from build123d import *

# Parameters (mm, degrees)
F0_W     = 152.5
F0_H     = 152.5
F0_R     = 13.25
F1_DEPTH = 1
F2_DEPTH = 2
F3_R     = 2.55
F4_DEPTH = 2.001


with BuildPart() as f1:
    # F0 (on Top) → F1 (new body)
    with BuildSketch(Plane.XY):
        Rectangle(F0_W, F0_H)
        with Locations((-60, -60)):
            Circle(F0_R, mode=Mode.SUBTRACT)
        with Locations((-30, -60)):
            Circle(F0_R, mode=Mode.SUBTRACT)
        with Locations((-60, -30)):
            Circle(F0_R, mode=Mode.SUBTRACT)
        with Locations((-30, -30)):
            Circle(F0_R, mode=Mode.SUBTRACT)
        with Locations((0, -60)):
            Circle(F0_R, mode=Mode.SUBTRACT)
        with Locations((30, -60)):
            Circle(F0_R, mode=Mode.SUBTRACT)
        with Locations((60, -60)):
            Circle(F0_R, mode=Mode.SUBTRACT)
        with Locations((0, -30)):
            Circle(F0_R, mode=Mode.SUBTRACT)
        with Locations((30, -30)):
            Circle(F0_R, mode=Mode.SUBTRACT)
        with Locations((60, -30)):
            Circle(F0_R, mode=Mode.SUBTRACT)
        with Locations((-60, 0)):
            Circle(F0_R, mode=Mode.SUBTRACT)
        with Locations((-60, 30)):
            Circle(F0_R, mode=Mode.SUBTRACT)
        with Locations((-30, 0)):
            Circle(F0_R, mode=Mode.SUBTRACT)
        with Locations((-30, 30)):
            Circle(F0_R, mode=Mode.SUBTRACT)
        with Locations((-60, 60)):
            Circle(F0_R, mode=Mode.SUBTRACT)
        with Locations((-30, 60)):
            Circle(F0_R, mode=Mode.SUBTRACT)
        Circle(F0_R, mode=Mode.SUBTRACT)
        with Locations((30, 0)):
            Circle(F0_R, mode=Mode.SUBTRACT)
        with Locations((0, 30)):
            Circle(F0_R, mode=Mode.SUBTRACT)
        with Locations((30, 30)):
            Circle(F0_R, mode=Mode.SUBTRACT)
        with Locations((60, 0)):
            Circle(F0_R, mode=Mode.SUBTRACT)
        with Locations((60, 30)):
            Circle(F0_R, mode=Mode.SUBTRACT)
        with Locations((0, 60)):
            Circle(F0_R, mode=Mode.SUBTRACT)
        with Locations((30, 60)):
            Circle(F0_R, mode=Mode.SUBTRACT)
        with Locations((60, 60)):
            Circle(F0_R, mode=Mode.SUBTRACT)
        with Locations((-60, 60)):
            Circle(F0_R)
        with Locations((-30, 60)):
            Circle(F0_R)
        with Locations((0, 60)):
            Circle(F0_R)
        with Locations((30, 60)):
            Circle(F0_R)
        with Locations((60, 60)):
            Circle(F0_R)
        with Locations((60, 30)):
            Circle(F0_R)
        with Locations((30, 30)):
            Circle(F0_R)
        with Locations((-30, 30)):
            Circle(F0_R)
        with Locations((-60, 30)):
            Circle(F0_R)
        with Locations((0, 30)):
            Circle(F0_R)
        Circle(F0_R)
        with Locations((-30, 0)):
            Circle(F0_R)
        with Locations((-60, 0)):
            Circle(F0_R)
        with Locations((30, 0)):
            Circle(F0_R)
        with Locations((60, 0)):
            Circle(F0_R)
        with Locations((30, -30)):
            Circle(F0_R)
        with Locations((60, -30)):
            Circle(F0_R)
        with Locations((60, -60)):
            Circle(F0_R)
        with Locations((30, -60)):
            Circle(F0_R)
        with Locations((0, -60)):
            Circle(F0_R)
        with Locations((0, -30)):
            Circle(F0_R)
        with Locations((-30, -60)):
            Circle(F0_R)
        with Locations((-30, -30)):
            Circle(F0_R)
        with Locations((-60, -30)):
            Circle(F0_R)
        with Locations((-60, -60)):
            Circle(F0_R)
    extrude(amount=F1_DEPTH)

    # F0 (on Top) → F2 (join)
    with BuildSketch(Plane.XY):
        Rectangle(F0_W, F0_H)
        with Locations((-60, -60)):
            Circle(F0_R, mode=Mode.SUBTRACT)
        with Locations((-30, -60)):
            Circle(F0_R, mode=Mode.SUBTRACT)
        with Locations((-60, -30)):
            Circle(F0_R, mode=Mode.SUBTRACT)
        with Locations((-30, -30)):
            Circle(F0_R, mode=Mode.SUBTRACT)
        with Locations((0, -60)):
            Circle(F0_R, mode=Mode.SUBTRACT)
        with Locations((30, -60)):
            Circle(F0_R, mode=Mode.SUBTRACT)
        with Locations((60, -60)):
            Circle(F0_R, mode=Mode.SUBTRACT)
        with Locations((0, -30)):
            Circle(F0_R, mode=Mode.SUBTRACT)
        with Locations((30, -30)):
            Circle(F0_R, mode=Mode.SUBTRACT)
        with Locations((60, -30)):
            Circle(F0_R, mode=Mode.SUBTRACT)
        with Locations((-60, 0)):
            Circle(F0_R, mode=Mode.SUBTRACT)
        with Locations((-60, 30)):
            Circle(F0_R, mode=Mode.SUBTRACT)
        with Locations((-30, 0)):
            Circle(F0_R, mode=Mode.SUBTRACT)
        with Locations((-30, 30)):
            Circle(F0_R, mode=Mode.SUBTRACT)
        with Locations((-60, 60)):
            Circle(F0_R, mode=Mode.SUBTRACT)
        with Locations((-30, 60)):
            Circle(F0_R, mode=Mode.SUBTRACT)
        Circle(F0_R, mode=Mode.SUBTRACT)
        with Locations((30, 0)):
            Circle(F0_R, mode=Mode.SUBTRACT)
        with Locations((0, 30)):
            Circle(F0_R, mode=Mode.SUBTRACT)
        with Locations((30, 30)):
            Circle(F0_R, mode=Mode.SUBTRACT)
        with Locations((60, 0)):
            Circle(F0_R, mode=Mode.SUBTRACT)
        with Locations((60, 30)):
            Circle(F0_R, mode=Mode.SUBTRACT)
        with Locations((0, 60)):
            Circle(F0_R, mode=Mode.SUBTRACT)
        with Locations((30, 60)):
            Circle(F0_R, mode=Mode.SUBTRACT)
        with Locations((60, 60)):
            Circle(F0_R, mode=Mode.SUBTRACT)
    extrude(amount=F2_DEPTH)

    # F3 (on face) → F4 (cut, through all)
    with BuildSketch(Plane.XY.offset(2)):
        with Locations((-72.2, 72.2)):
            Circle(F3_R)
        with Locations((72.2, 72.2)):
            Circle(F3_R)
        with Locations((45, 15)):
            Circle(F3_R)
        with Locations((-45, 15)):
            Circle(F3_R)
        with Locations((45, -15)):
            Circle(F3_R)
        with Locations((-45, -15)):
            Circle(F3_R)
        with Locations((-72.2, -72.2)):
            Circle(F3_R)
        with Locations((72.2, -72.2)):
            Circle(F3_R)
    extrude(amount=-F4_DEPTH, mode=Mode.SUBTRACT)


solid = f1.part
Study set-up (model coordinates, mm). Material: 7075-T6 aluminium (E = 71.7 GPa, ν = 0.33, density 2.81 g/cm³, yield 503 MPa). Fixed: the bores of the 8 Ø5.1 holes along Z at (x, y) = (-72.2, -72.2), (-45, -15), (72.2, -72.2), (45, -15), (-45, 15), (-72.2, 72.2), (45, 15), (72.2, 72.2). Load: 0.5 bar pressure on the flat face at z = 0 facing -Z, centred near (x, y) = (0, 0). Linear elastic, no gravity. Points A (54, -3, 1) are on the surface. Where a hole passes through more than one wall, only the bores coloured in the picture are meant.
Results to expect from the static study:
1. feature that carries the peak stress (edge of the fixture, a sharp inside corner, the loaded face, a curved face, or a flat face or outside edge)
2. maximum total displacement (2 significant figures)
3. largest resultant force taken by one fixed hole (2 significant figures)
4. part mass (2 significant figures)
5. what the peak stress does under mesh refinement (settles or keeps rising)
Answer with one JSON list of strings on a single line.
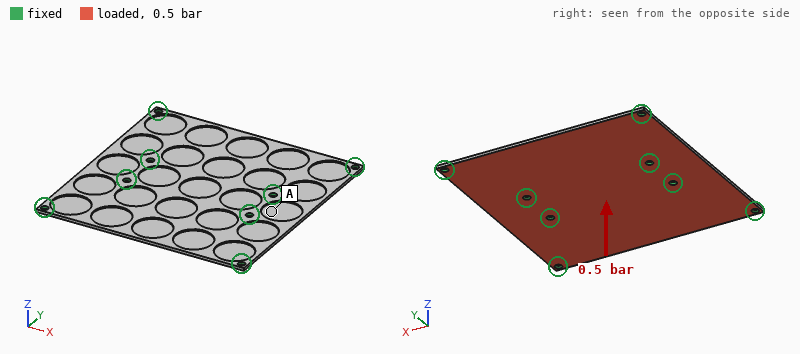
["edge of the fixture", "1.7 mm", "260 N", "91 g", "keeps rising"]
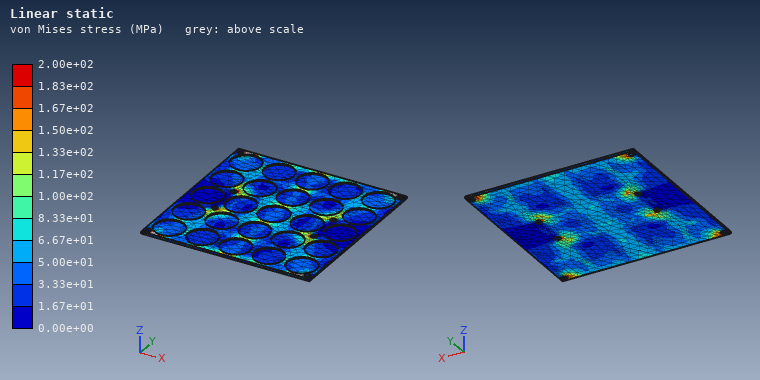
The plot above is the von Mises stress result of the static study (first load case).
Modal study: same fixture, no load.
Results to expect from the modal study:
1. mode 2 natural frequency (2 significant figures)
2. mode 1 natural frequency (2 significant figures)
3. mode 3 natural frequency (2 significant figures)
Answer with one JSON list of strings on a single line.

["570 Hz", "560 Hz", "1200 Hz"]
